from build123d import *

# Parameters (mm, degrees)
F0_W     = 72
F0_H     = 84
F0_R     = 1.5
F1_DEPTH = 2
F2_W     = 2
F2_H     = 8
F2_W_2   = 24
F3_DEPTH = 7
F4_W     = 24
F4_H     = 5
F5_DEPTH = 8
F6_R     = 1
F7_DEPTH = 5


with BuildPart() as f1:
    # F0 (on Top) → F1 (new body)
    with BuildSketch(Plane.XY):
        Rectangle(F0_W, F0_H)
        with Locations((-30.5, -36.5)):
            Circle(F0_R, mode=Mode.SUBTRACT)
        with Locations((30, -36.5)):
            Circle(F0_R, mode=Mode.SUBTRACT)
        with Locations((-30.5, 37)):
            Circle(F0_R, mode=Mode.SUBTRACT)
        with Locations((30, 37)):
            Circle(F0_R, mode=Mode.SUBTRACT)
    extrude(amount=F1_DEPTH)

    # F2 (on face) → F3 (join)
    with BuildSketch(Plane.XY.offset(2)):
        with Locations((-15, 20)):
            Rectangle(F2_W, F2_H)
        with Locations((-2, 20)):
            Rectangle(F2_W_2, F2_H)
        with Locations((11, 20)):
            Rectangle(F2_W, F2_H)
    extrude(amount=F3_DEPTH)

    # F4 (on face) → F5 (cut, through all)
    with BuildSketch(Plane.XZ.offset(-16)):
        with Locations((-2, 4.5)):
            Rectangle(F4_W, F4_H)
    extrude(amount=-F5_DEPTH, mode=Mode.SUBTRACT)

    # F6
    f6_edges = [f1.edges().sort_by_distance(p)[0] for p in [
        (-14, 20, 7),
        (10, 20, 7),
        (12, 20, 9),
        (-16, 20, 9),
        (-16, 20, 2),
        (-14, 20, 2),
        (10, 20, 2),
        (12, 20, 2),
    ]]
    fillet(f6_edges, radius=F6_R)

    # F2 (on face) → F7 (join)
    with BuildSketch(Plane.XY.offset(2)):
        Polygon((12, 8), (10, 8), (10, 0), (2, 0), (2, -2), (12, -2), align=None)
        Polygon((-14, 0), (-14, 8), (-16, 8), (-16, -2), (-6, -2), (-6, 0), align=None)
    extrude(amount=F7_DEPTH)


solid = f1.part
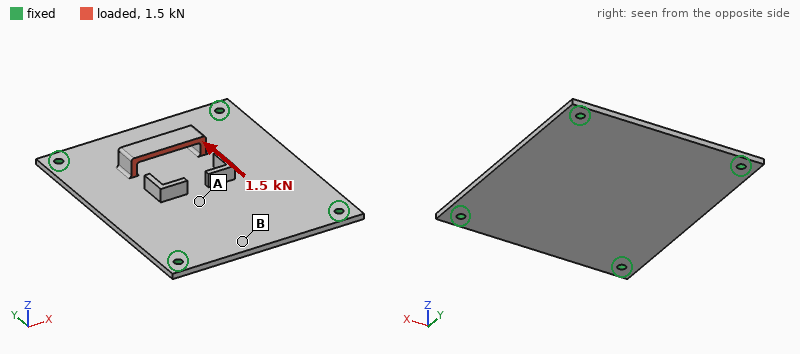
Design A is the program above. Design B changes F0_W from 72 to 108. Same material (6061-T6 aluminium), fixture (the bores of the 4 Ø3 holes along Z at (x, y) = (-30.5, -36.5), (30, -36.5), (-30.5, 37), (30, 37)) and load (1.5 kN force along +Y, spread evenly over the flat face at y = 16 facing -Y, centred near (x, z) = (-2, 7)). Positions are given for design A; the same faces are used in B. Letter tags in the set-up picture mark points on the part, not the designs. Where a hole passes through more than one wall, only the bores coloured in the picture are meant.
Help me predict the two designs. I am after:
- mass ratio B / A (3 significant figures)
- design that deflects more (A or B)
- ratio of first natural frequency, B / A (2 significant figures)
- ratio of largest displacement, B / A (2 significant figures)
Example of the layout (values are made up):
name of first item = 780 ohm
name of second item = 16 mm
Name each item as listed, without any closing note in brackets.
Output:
mass ratio B / A = 1.46
design that deflects more = A
ratio of first natural frequency, B / A = 1.0
ratio of largest displacement, B / A = 0.91
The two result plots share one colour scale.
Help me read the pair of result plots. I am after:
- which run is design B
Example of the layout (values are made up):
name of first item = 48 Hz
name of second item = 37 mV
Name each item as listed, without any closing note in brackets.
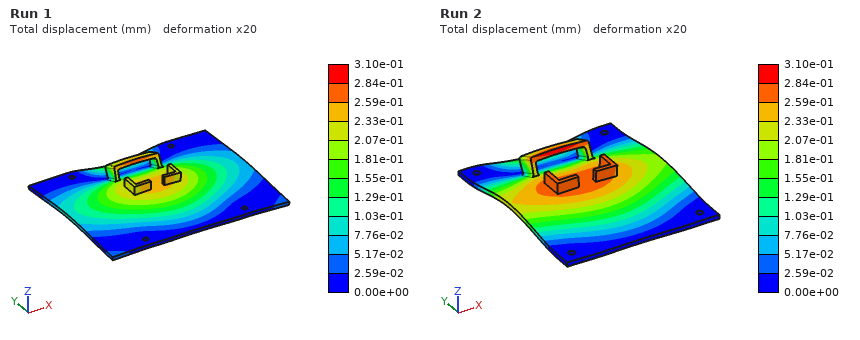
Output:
which run is design B = Run 1
